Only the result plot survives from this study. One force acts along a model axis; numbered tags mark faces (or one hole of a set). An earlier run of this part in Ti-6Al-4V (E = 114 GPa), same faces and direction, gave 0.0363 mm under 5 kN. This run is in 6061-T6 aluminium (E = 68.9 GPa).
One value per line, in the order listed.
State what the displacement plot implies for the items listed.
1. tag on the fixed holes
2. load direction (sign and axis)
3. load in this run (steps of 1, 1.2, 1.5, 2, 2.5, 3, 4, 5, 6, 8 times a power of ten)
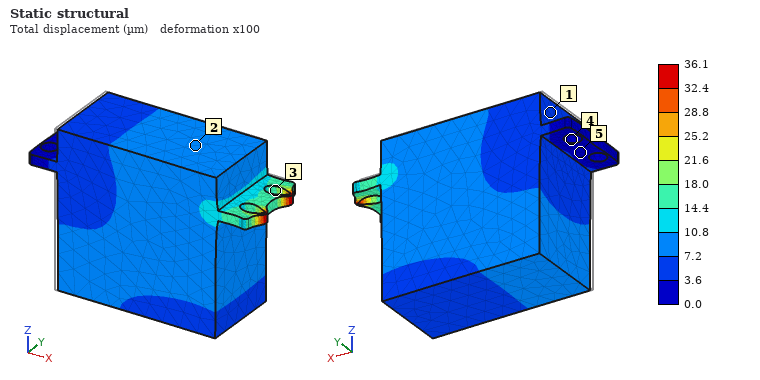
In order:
4
+X
3 kN
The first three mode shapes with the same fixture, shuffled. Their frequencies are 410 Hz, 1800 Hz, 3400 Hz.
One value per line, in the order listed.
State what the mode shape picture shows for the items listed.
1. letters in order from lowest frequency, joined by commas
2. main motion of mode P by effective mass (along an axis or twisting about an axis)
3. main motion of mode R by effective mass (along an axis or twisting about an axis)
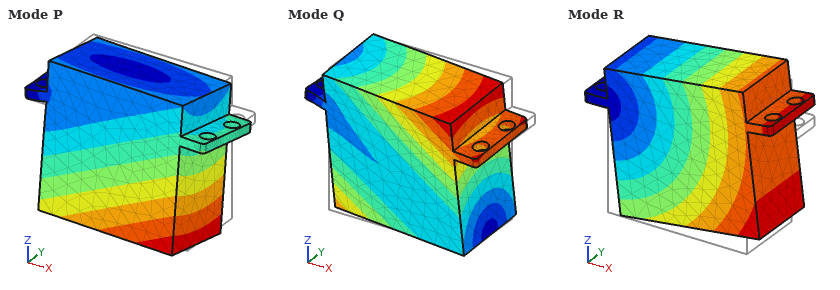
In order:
R, P, Q
along Y
along Z
